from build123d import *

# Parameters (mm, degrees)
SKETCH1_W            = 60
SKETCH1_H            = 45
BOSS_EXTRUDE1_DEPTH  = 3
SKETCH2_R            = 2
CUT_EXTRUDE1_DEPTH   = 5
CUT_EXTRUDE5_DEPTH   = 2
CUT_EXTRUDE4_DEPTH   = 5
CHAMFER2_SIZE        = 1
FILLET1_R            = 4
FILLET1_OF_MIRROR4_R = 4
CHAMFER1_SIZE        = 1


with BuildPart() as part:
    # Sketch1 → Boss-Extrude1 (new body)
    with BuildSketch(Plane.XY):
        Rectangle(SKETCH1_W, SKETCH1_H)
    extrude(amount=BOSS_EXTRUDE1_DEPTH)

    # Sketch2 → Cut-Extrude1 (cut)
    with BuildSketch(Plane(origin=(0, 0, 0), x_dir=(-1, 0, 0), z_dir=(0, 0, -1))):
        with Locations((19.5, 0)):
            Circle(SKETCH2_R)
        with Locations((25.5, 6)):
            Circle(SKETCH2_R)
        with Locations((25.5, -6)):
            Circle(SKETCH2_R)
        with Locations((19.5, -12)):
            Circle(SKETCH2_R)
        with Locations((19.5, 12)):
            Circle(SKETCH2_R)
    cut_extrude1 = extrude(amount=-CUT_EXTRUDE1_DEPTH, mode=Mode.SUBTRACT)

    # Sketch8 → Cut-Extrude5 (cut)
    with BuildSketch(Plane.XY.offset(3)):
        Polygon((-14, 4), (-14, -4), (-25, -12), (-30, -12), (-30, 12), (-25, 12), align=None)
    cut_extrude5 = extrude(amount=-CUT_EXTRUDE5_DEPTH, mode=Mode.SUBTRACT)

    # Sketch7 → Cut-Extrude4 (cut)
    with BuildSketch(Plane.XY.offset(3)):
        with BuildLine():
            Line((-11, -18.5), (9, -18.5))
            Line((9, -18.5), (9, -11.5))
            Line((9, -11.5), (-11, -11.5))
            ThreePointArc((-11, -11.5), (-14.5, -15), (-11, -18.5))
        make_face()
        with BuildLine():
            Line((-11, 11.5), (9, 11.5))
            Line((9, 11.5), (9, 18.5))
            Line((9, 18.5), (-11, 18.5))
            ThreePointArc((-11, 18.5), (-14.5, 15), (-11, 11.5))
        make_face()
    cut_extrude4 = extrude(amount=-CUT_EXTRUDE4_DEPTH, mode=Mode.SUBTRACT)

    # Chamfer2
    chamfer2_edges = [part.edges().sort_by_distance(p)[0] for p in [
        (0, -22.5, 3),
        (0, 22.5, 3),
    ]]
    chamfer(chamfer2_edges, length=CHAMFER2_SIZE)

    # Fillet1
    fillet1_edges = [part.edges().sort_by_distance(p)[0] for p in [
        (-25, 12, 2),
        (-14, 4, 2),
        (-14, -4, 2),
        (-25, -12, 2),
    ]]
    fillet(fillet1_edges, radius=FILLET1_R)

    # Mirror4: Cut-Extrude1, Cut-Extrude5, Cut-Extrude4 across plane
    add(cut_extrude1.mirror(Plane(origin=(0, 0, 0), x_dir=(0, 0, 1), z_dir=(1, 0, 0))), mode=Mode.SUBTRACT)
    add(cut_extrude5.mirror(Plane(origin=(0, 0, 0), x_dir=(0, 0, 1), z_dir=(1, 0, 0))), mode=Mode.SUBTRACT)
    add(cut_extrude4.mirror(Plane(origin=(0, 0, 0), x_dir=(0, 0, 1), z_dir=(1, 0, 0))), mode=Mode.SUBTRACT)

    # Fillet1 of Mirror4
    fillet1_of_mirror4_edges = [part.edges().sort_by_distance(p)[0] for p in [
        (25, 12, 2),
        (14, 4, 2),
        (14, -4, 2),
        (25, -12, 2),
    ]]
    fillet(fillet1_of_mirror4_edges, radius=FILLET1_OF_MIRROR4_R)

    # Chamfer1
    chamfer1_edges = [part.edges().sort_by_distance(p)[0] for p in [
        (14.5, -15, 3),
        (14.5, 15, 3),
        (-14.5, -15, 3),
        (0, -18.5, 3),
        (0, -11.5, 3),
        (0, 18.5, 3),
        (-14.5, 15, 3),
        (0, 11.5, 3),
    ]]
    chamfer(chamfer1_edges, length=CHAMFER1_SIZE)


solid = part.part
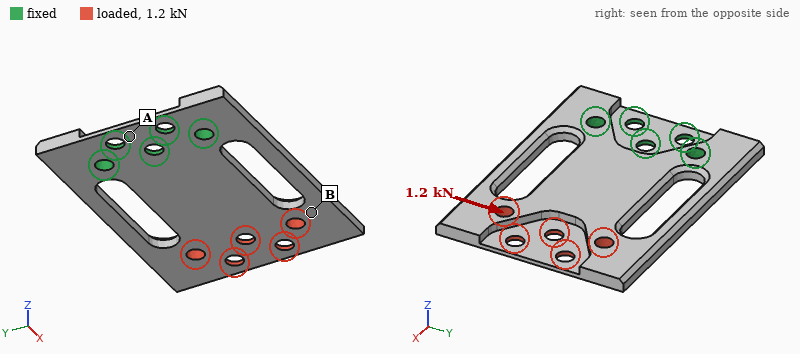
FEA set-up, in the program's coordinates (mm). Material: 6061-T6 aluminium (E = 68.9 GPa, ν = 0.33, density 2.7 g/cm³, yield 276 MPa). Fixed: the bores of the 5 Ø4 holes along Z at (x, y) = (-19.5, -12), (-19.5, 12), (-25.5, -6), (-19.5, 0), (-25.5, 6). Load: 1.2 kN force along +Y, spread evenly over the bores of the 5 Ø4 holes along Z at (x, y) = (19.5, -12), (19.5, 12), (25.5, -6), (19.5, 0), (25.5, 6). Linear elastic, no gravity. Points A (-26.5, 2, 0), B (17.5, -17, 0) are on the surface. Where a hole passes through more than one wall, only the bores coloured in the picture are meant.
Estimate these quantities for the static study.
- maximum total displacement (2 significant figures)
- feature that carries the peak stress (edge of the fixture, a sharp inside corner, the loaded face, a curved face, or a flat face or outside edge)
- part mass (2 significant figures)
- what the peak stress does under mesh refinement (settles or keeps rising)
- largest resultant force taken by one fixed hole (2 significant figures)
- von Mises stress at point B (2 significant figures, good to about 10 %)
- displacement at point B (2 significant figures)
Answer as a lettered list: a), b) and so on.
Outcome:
a) 0.11 mm
b) a sharp inside corner
c) 15 g
d) keeps rising
e) 1.9 kN
f) 39 MPa
g) 0.084 mm
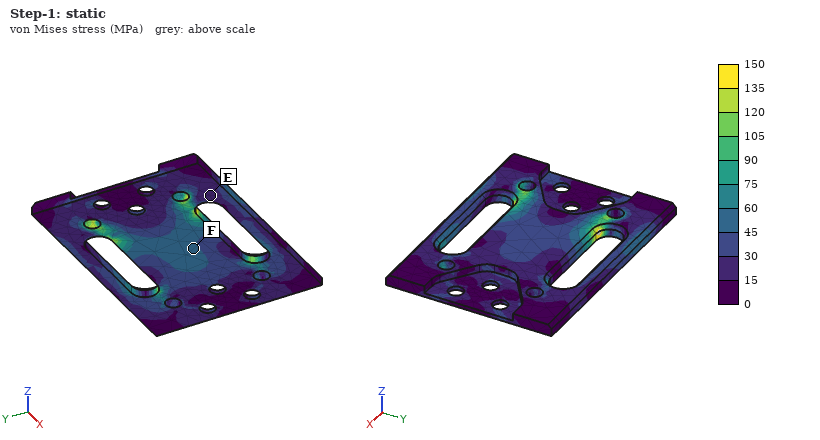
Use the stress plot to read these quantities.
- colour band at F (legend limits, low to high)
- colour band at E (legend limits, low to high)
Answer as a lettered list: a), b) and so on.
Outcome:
a) 45 to 60 MPa
b) 15 to 30 MPa
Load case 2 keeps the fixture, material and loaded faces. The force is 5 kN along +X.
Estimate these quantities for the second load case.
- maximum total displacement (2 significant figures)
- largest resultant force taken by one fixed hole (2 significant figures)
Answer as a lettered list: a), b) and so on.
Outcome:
a) 0.28 mm
b) 2.0 kN
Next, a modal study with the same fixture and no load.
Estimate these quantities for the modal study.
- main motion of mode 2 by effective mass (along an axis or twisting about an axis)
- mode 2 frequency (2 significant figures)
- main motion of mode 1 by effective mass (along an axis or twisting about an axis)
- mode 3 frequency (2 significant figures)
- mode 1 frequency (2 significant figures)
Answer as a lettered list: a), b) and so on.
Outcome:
a) twisting about X
b) 2100 Hz
c) along Z
d) 5700 Hz
e) 980 Hz
